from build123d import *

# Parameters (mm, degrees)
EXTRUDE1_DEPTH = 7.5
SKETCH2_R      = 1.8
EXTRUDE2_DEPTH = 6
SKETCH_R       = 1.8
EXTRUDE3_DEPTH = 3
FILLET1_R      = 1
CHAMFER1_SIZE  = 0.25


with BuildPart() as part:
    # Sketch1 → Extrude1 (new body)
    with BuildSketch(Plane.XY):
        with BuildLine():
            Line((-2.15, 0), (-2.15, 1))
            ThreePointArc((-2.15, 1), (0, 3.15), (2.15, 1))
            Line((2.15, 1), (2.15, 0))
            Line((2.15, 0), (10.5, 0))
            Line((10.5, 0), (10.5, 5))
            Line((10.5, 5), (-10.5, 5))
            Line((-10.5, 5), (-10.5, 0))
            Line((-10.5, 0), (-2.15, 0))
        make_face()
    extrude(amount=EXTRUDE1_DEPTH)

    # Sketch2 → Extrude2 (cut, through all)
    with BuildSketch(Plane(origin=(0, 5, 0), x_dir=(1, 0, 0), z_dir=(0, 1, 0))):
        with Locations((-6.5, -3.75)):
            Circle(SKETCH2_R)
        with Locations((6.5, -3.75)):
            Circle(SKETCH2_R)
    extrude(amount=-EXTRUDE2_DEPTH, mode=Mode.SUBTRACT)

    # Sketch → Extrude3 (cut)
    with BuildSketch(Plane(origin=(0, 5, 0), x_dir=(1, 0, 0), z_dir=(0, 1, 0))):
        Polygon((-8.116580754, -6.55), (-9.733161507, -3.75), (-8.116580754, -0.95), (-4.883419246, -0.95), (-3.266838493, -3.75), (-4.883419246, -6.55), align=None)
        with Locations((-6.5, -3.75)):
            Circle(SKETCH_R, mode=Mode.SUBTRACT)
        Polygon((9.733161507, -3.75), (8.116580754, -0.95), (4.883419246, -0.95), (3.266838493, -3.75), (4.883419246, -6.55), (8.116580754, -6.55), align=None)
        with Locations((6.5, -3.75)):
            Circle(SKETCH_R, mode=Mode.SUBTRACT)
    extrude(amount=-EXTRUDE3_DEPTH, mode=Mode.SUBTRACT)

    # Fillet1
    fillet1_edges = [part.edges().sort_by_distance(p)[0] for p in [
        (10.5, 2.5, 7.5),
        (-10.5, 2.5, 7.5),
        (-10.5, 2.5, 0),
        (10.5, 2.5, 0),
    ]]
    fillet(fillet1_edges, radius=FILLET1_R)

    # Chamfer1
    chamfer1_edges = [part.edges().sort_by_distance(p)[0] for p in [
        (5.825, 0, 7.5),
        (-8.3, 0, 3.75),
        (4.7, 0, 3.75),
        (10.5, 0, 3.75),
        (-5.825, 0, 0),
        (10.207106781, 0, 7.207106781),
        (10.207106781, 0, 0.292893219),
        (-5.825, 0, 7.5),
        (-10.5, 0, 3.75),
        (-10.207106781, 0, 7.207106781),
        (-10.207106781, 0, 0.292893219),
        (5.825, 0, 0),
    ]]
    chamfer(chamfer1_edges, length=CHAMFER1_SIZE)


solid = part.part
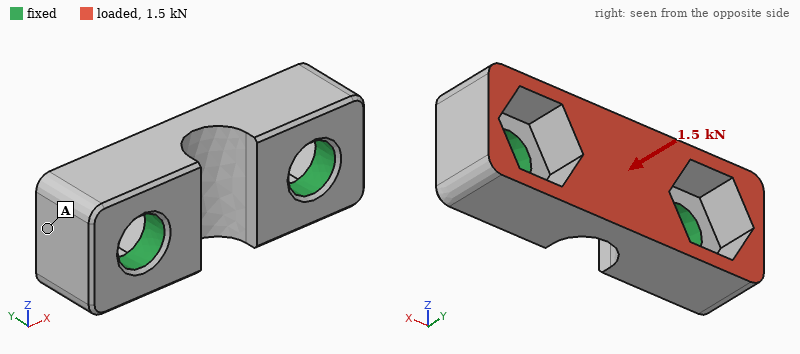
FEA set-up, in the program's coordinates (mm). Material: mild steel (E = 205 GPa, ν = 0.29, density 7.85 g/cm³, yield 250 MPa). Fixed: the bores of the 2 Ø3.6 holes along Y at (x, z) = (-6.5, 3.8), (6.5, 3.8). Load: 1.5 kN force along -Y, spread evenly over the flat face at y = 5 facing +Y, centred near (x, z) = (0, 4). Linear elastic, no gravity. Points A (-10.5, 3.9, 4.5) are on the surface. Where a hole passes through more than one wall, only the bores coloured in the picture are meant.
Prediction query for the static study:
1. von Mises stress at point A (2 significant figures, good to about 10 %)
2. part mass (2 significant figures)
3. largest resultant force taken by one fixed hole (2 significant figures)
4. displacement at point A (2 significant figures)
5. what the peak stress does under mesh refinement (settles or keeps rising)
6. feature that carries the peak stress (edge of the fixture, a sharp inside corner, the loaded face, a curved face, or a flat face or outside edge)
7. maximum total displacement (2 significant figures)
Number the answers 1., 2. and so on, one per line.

1. 19 MPa
2. 3.9 g
3. 800 N
4. 0.70 µm
5. keeps rising
6. edge of the fixture
7. 2.2 µm
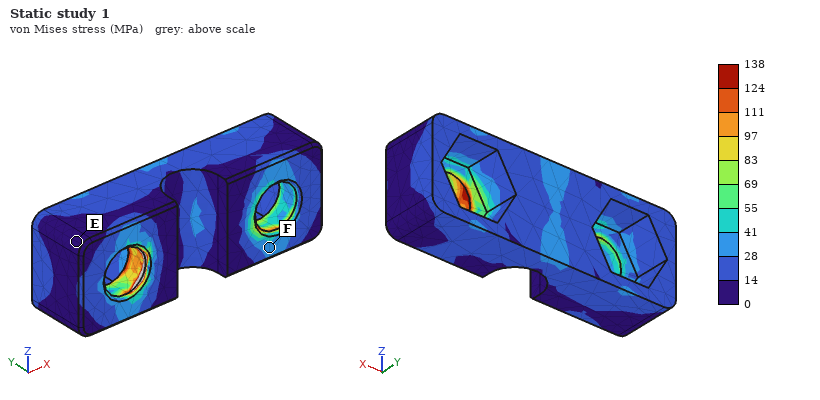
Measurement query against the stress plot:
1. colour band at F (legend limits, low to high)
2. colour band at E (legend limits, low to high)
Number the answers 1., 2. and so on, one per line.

1. 28 to 41 MPa
2. 0 to 14 MPa
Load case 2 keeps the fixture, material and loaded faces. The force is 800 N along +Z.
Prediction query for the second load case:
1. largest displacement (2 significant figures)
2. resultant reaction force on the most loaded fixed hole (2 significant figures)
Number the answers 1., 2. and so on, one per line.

1. 5.7 µm
2. 400 N
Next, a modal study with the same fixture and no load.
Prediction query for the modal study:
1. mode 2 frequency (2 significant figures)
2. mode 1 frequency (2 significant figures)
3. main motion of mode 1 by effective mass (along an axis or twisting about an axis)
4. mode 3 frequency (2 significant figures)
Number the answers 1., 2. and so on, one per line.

1. 77 kHz
2. 55 kHz
3. along Z
4. 79 kHz
